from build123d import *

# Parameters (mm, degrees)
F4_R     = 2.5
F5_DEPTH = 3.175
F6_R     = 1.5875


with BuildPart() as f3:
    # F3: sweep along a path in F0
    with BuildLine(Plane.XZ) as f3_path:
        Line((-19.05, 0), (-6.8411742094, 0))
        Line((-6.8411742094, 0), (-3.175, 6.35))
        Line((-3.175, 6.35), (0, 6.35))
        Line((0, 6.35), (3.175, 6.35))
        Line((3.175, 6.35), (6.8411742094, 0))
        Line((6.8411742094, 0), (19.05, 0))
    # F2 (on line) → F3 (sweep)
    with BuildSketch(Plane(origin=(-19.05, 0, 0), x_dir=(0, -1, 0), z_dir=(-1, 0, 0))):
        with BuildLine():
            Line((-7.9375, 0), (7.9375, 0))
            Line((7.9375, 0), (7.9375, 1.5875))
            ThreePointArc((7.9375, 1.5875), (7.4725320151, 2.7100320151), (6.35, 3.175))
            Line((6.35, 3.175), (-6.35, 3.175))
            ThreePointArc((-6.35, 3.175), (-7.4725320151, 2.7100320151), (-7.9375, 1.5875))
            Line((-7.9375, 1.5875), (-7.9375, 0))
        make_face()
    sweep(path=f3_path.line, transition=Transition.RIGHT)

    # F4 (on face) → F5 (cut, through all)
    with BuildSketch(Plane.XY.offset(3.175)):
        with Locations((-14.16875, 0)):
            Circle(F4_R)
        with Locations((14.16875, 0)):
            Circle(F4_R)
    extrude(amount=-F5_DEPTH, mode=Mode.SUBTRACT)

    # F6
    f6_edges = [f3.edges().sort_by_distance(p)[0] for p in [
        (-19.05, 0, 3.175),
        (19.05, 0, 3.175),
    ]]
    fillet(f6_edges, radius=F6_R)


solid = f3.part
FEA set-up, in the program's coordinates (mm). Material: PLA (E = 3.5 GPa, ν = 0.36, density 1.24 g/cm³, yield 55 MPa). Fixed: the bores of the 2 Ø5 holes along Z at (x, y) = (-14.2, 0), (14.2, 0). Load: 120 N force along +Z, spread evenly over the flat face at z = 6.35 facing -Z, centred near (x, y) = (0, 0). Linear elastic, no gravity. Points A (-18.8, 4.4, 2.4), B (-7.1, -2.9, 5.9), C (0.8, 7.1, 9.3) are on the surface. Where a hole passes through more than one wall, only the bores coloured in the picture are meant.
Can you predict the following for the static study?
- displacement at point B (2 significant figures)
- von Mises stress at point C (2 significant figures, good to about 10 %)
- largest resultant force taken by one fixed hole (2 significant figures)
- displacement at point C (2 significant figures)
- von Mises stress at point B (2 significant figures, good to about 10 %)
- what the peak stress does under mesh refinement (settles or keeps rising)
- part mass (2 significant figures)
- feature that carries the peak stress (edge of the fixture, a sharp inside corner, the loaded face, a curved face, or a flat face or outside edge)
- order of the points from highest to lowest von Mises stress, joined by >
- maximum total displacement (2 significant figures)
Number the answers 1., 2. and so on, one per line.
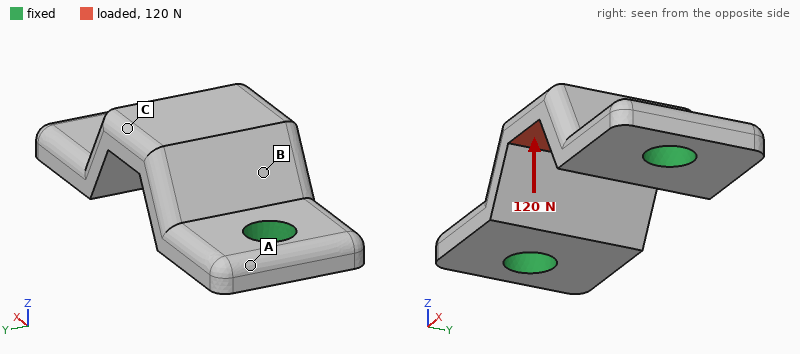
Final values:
1. 17 µm
2. 4.4 MPa
3. 88 N
4. 26 µm
5. 2.5 MPa
6. keeps rising
7. 2.6 g
8. edge of the fixture
9. C > B > A
10. 28 µm
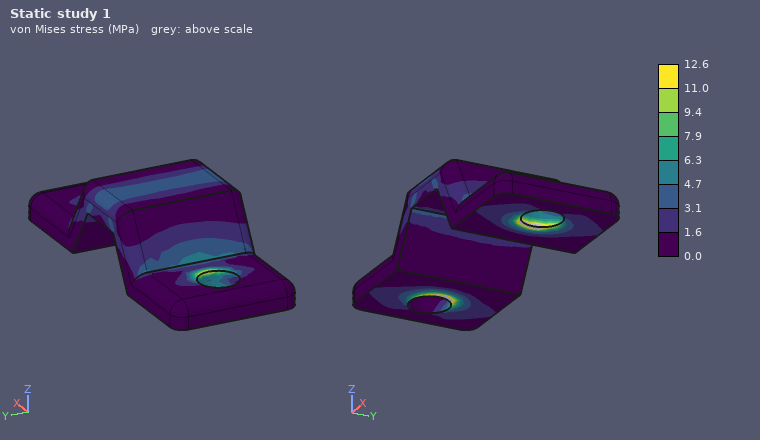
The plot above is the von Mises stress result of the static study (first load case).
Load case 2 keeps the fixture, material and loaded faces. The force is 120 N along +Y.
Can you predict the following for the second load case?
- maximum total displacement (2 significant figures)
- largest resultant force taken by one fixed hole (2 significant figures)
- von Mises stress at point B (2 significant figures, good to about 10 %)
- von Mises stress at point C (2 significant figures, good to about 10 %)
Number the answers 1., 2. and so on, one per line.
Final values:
1. 83 µm
2. 60 N
3. 4.5 MPa
4. 2.3 MPa
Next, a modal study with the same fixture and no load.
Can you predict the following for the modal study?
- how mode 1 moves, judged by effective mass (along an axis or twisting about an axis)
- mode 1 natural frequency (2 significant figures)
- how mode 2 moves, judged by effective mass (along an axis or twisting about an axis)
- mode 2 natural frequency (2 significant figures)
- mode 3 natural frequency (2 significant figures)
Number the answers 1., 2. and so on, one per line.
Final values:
1. along Y
2. 5500 Hz
3. along Z
4. 9900 Hz
5. 13 kHz
